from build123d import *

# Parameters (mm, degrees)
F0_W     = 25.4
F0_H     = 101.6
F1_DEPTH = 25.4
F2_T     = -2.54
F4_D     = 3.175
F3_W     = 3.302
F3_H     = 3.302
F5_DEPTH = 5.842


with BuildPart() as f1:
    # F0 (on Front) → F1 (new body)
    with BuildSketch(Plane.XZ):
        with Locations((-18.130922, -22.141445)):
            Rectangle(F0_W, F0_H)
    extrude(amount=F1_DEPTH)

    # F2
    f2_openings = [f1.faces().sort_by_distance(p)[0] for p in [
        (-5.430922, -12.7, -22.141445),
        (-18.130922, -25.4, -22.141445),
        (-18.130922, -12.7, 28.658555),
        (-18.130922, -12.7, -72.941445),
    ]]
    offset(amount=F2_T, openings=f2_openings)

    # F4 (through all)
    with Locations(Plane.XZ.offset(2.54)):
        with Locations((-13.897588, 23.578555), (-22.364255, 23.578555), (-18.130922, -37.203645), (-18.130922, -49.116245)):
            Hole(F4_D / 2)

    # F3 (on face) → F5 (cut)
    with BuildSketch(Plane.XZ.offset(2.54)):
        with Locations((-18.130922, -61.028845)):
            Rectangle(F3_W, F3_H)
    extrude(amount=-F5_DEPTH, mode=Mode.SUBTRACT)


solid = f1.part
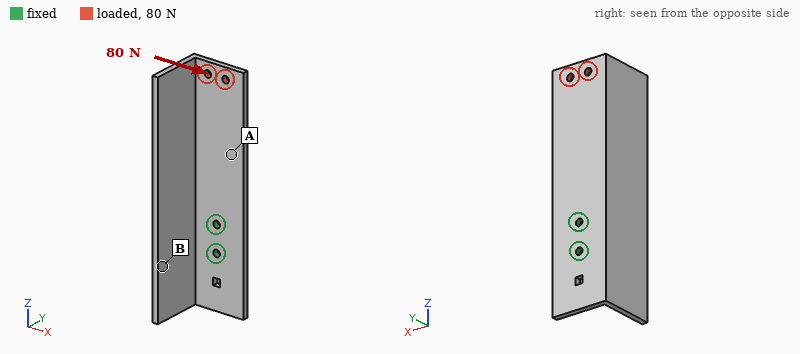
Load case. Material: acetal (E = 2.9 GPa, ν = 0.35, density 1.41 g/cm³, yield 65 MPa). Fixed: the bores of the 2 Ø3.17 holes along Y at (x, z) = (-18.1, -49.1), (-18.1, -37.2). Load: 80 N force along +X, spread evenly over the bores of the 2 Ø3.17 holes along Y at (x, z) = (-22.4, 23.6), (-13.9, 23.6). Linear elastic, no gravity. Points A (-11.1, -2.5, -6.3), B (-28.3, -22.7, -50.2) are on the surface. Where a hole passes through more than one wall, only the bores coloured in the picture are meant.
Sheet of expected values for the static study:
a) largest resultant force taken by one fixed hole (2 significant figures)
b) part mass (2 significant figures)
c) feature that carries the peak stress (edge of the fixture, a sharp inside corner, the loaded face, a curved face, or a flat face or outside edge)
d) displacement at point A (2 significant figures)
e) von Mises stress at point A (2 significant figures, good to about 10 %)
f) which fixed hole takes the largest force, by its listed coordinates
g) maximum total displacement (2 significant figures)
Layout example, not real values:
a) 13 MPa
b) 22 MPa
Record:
a) 400 N
b) 17 g
c) edge of the fixture
d) 0.47 mm
e) 5.1 MPa
f) (-18.1, -37.2)
g) 1.2 mm
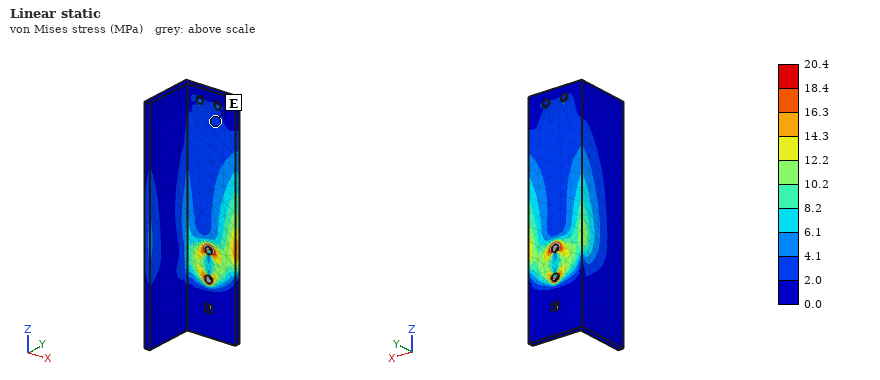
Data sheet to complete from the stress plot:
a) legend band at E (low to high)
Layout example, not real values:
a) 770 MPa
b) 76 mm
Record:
a) 2.0 to 4.1 MPa
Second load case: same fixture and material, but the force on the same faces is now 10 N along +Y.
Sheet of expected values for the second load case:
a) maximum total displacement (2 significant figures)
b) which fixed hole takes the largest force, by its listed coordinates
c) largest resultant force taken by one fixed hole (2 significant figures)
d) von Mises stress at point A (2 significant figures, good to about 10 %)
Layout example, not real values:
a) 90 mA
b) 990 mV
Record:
a) 1.2 mm
b) (-18.1, -37.2)
c) 41 N
d) 1.9 MPa
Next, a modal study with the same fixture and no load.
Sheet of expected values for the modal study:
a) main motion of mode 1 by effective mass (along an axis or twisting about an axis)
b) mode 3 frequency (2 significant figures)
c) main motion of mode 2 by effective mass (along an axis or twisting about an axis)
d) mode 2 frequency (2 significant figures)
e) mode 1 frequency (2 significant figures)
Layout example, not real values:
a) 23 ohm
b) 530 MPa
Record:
a) along Y
b) 620 Hz
c) along X
d) 340 Hz
e) 250 Hz
